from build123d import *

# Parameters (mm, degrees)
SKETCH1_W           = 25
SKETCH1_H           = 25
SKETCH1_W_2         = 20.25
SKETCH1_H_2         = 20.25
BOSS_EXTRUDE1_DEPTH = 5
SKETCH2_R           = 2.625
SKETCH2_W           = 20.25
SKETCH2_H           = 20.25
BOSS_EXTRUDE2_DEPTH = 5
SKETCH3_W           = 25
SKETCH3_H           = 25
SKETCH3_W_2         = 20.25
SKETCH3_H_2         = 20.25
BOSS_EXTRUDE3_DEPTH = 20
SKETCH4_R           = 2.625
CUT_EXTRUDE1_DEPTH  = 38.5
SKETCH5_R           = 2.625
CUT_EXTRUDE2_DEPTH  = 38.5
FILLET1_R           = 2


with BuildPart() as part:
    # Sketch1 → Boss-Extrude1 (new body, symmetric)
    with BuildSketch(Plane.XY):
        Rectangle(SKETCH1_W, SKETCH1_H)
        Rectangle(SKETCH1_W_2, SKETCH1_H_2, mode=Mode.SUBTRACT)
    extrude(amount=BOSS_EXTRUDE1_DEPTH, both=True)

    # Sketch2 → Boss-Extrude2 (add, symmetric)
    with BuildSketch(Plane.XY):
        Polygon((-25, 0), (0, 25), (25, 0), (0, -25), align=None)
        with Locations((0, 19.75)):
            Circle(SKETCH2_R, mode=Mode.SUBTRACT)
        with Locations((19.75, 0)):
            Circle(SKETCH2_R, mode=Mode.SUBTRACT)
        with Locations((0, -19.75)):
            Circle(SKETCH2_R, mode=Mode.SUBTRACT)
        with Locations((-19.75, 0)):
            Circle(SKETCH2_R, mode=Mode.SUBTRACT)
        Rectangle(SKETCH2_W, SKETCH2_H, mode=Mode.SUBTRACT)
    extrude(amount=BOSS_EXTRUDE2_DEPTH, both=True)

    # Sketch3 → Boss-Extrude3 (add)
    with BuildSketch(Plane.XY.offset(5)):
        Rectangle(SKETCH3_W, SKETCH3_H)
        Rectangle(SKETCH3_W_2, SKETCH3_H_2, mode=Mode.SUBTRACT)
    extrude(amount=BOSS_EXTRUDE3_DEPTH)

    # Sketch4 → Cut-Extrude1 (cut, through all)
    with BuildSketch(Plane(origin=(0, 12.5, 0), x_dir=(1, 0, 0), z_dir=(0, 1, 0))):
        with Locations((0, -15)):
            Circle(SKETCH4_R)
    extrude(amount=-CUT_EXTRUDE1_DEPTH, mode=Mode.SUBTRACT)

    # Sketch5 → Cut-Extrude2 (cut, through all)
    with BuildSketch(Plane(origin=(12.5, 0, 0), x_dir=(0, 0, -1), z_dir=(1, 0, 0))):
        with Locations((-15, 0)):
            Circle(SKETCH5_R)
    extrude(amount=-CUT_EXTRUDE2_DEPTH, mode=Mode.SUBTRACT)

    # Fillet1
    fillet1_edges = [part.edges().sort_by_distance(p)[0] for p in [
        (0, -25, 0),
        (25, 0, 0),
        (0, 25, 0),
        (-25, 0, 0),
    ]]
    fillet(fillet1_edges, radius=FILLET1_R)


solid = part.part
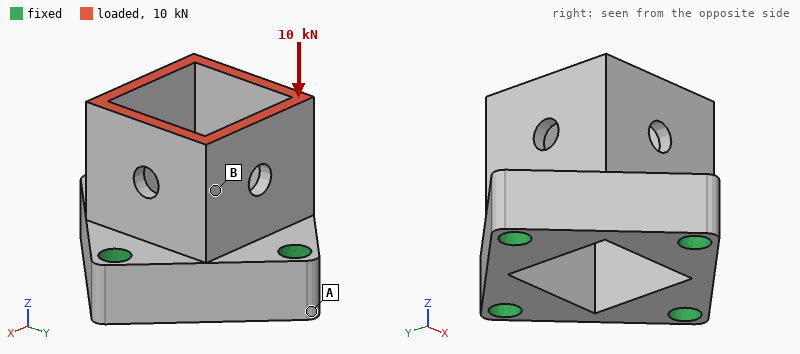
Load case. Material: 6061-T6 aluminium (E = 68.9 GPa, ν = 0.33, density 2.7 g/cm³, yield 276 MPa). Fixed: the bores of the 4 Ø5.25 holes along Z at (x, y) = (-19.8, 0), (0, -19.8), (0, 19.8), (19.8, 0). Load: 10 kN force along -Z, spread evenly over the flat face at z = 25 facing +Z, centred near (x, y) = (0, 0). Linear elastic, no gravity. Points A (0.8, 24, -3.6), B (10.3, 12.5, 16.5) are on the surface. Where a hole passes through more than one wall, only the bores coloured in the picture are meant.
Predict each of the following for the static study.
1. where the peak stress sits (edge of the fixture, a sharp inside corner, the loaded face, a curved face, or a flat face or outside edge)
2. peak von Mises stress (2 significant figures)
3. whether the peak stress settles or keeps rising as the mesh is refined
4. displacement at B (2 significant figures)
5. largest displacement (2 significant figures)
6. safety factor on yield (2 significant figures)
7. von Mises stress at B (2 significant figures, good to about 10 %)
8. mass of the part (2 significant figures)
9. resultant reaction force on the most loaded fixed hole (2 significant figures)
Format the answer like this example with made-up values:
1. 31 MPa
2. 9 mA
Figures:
1. a curved face
2. 160 MPa
3. settles
4. 18 µm
5. 26 µm
6. 1.7
7. 41 MPa
8. 31 g
9. 2.5 kN
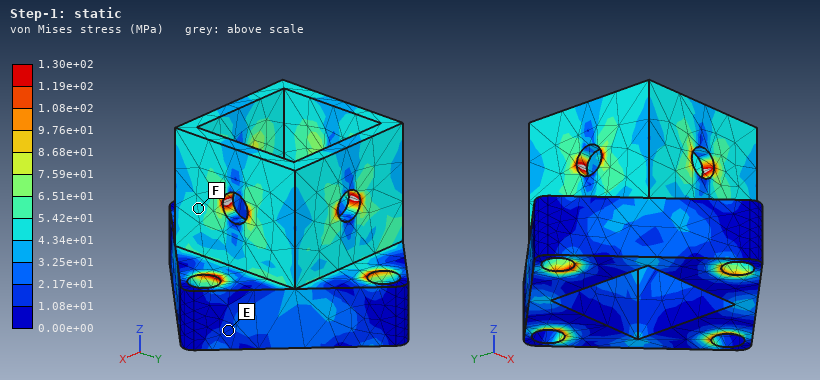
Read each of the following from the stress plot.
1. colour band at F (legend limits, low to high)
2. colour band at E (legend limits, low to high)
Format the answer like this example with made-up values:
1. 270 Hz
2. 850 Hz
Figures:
1. 4.34e+01 to 5.42e+01 MPa
2. 1.08e+01 to 2.17e+01 MPa
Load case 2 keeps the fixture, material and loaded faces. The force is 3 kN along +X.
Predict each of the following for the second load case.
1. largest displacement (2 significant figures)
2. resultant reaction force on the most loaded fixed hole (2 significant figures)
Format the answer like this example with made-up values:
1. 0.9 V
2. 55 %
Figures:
1. 0.14 mm
2. 2.1 kN
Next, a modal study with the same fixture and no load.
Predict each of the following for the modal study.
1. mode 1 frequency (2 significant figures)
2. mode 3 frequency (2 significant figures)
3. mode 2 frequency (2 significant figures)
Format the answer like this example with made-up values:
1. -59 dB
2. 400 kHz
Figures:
1. 14 kHz
2. 16 kHz
3. 15 kHz
